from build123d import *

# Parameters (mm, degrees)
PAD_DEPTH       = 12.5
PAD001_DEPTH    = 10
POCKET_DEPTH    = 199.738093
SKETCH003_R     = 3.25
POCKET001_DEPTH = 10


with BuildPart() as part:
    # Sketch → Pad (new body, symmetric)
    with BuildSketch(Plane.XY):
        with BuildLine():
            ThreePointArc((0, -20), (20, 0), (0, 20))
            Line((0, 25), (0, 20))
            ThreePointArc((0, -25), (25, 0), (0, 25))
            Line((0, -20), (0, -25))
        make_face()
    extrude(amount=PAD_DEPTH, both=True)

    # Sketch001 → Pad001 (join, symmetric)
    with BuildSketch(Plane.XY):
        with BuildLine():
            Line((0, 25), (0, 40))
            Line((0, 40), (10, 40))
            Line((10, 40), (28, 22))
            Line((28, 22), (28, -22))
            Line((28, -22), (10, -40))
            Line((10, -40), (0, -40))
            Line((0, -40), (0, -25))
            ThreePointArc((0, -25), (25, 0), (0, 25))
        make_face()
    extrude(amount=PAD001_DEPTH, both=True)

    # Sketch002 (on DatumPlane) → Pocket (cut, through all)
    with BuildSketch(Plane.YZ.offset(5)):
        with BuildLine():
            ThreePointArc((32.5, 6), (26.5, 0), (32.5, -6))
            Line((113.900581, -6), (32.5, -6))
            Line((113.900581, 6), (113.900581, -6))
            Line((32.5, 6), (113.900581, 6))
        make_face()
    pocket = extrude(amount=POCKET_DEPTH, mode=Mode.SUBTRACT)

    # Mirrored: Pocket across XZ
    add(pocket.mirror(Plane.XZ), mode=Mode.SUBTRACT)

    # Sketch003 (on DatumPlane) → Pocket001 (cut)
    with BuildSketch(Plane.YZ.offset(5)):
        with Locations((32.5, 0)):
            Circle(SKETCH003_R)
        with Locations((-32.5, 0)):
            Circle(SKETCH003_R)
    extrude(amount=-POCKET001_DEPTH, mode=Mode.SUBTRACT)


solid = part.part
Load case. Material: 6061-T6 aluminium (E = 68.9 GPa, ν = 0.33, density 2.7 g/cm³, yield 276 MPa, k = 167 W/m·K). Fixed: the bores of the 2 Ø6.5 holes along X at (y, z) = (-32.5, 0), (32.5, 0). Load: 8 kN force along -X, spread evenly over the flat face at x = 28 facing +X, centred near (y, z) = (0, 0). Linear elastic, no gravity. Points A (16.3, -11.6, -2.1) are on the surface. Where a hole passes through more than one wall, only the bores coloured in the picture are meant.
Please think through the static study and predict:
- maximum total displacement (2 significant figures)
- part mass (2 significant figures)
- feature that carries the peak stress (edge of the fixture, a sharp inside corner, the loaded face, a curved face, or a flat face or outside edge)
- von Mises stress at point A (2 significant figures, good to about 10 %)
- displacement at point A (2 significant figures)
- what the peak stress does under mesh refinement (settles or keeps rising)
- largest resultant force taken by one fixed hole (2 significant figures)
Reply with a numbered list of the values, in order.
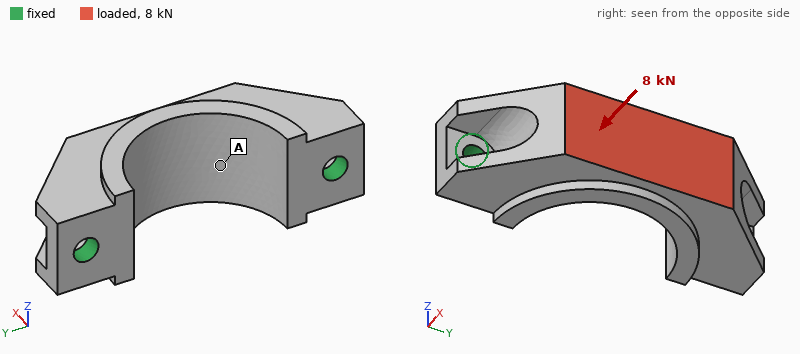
1. 31 µm
2. 65 g
3. edge of the fixture
4. 27 MPa
5. 23 µm
6. keeps rising
7. 5.2 kN
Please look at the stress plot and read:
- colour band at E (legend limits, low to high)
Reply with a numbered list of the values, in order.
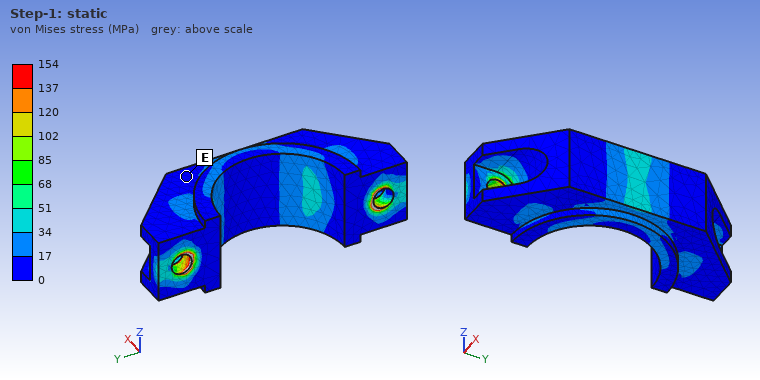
1. 0 to 17 MPa
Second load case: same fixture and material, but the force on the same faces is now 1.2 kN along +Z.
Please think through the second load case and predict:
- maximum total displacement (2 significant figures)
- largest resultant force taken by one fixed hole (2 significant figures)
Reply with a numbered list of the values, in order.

1. 60 µm
2. 600 N
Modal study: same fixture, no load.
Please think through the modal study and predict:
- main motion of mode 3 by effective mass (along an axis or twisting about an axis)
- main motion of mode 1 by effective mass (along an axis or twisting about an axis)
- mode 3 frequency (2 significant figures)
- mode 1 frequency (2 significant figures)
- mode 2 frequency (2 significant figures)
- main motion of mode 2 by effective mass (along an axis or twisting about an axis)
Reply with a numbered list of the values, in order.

1. along Y
2. along Z
3. 11 kHz
4. 4600 Hz
5. 11 kHz
6. twisting about X
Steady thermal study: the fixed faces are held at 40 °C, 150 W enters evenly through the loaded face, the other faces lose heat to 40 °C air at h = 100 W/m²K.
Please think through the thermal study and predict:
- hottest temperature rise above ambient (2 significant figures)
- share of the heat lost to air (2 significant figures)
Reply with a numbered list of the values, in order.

1. 59 K
2. 14 %
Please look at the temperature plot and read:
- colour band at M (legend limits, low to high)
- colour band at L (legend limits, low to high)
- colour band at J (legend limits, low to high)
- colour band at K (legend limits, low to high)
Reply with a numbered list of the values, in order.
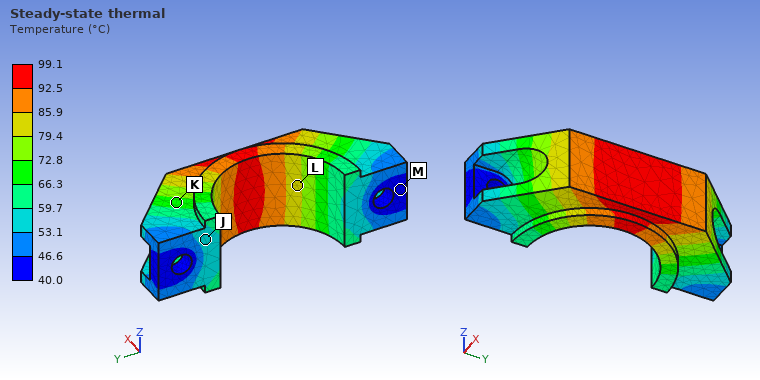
1. 40.0 to 46.6 °C
2. 79.4 to 85.9 °C
3. 53.1 to 59.7 °C
4. 66.3 to 72.8 °C
